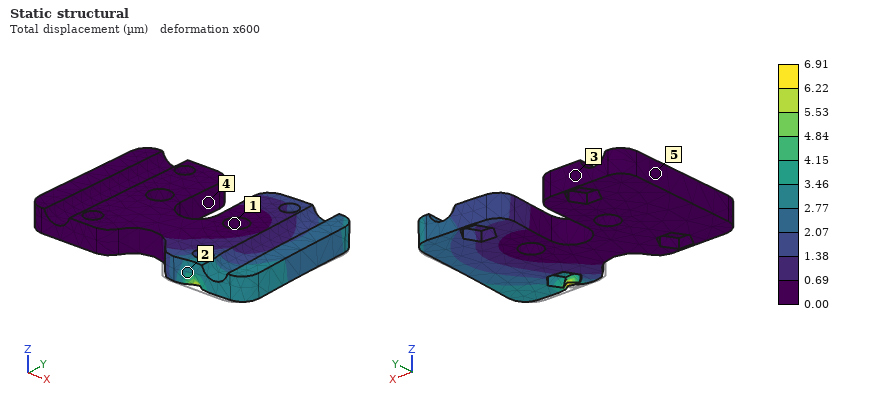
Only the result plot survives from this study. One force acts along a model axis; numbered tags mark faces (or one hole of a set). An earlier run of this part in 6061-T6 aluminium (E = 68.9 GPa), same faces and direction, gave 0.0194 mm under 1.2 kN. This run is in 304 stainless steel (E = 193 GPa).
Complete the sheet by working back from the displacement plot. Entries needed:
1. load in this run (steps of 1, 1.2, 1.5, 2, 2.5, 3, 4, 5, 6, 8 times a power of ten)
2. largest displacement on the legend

1.2 kN
6.91 µm
